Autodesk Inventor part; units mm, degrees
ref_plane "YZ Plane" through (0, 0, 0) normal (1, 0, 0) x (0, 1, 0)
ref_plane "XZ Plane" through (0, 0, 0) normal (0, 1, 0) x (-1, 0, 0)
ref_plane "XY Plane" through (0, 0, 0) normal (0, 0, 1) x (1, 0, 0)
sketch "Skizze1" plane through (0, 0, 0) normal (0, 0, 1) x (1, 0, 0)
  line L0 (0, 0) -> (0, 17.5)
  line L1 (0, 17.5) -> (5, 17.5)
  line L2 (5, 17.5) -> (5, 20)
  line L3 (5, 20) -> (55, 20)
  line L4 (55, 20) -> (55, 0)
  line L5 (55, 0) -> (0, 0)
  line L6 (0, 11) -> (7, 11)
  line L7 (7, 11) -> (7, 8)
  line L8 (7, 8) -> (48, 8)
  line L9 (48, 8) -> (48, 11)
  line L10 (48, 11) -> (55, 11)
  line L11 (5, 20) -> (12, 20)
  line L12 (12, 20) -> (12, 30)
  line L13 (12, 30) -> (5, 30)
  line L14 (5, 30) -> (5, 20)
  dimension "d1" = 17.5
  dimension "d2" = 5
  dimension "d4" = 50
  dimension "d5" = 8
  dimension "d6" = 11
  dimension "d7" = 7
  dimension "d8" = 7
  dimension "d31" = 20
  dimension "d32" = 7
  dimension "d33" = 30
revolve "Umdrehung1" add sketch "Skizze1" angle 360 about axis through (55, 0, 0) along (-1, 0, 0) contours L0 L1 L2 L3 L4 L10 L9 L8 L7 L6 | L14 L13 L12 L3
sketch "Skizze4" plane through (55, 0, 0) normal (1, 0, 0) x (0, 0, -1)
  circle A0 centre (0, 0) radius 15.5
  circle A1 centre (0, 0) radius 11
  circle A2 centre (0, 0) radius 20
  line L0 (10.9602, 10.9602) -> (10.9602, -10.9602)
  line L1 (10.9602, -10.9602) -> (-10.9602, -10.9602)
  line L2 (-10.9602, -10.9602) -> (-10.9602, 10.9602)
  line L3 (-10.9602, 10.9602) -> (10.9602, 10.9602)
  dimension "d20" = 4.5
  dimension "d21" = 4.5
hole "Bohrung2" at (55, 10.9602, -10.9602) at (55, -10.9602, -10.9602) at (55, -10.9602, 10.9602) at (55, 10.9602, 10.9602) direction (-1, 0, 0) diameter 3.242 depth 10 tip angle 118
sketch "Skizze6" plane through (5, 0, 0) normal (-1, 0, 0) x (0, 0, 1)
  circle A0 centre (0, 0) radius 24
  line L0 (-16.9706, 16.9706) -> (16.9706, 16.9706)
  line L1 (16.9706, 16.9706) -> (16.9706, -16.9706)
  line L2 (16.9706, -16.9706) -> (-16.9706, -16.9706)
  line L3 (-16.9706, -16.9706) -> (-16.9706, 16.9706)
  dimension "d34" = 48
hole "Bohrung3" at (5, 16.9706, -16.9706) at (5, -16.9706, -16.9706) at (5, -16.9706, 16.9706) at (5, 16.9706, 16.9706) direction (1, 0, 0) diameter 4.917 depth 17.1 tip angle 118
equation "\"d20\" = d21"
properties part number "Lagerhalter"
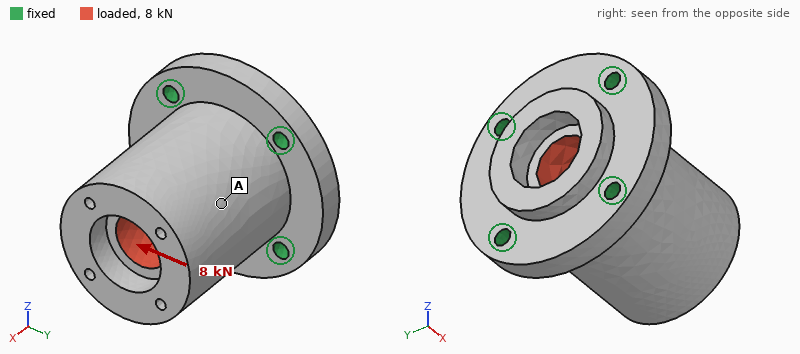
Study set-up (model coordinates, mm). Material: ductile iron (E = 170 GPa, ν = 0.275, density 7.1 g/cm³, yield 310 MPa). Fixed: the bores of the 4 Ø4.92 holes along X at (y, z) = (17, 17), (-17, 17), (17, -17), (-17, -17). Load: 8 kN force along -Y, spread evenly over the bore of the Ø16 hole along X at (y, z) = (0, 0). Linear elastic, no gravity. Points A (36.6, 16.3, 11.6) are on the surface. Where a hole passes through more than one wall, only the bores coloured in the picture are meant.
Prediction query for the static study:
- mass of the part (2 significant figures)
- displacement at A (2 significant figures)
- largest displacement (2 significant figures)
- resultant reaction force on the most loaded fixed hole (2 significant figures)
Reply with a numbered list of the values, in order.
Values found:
1. 460 g
2. 9.7 µm
3. 14 µm
4. 3.1 kN
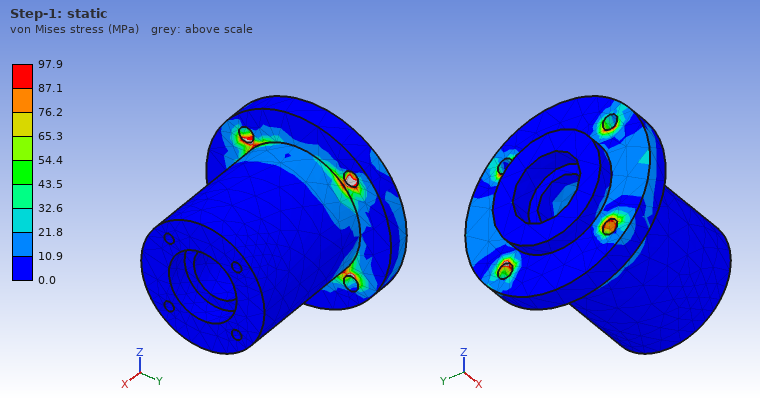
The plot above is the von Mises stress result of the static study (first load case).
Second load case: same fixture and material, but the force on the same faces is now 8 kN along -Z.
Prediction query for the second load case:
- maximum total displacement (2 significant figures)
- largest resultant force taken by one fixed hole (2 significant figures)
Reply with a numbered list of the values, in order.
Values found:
1. 14 µm
2. 3.1 kN
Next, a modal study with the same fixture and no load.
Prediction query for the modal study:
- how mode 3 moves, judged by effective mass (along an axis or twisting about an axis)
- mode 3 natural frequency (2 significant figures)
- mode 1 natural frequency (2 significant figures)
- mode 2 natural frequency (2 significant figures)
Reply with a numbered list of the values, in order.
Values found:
1. along X
2. 13 kHz
3. 6900 Hz
4. 6900 Hz
